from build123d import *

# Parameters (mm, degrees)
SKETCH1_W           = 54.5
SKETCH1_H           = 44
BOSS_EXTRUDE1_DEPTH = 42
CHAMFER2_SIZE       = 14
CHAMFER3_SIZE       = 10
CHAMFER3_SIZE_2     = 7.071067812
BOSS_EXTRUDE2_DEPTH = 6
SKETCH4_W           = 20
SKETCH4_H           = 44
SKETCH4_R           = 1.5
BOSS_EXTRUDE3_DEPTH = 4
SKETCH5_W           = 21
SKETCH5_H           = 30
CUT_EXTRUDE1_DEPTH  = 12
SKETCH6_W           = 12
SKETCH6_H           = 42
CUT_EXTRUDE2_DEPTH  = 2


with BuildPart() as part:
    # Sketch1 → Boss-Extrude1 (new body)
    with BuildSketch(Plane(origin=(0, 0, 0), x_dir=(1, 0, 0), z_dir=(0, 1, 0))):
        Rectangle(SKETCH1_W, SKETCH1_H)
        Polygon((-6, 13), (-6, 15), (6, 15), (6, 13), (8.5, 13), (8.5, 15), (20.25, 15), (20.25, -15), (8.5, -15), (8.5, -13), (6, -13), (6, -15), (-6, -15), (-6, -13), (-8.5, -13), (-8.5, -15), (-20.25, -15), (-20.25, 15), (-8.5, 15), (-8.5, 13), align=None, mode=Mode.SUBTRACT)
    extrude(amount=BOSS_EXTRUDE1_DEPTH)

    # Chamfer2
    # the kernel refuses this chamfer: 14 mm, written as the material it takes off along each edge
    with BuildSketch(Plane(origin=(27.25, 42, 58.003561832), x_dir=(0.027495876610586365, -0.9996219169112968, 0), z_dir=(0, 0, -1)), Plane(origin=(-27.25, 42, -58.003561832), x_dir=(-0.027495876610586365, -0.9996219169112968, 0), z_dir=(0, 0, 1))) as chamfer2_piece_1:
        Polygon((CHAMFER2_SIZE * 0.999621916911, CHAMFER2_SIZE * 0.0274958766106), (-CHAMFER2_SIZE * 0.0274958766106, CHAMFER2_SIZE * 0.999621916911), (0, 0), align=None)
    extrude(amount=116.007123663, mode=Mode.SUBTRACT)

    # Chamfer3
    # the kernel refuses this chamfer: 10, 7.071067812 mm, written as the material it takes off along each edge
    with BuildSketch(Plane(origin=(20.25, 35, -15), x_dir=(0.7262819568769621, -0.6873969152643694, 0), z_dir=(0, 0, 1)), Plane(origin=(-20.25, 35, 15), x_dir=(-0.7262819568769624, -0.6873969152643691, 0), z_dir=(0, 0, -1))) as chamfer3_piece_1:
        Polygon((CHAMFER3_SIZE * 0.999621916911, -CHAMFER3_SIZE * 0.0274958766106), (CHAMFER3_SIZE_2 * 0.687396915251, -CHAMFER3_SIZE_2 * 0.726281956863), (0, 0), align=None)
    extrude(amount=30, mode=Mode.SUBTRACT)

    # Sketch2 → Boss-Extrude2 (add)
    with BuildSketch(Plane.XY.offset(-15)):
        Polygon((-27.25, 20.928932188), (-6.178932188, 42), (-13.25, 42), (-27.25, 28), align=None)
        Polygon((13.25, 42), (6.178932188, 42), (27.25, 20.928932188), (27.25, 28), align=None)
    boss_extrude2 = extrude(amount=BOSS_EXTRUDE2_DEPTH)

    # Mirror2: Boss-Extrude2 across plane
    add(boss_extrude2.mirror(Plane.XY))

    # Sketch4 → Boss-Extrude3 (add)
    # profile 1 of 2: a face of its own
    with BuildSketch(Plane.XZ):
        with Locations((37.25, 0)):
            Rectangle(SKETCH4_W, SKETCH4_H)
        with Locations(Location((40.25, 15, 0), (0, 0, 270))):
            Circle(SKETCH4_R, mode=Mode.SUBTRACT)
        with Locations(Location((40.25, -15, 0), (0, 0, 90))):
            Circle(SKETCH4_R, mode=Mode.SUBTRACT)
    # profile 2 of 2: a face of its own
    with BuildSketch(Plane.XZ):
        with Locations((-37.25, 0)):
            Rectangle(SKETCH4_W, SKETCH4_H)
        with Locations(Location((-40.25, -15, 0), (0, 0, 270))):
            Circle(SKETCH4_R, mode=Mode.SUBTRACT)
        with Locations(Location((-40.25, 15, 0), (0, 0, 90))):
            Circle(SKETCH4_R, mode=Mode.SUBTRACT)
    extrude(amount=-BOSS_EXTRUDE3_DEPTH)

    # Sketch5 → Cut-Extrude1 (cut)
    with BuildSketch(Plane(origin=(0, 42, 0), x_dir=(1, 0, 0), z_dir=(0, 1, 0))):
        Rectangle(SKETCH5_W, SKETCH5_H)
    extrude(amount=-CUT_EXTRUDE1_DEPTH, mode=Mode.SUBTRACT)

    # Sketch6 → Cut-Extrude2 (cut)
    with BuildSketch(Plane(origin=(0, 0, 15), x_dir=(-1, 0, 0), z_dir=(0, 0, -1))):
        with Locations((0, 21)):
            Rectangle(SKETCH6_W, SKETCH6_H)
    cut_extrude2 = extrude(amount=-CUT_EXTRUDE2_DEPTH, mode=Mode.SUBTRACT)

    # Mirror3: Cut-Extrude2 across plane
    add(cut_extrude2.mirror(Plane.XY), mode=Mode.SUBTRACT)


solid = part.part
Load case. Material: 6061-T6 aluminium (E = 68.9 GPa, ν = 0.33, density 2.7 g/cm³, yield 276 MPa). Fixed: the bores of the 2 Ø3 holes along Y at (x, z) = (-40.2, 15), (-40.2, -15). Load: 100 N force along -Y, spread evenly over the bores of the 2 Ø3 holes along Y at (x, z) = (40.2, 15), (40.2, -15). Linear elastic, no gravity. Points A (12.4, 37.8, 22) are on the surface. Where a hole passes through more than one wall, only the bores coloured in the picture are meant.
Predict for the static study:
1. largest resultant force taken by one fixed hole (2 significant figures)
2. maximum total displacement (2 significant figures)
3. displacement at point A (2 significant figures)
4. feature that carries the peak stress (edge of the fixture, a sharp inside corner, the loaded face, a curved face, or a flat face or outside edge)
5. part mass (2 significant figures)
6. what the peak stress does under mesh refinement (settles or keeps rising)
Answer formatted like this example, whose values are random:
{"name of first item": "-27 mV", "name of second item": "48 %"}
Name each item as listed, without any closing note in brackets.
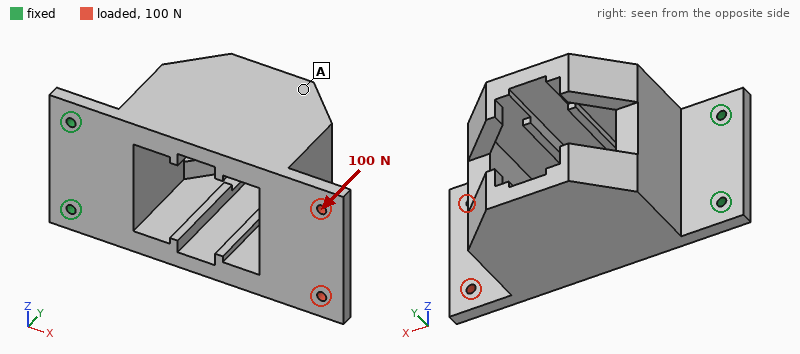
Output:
{"largest resultant force taken by one fixed hole": "65 N", "maximum total displacement": "0.63 mm", "displacement at point A": "0.44 mm", "feature that carries the peak stress": "edge of the fixture", "part mass": "130 g", "what the peak stress does under mesh refinement": "keeps rising"}
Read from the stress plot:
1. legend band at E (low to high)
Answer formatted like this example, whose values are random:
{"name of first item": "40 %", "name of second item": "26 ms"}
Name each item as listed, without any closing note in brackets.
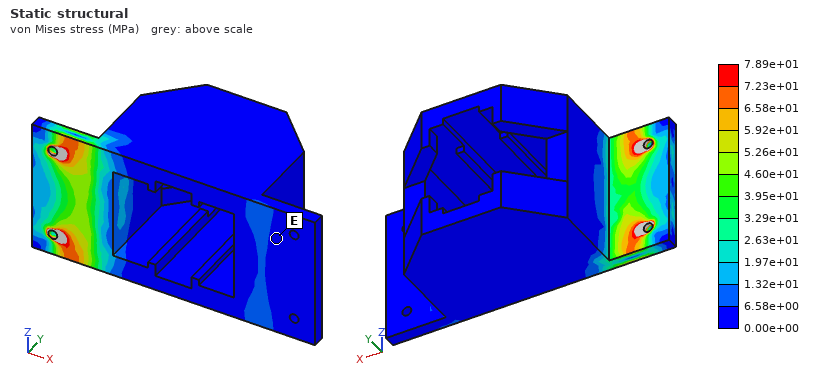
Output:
{"legend band at E": "0.00e+00 to 6.58e+00 MPa"}
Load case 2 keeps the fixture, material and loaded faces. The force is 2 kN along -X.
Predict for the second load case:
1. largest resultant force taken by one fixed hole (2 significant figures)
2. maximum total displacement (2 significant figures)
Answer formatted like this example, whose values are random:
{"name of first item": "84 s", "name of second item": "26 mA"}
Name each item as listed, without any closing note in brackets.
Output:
{"largest resultant force taken by one fixed hole": "1.0 kN", "maximum total displacement": "67 µm"}
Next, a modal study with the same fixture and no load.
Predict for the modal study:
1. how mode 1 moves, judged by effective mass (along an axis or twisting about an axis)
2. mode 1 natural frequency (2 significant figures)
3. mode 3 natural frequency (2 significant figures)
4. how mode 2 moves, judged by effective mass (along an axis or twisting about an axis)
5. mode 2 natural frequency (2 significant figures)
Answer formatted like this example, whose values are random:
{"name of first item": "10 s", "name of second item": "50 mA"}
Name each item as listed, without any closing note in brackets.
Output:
{"how mode 1 moves, judged by effective mass": "along Y", "mode 1 natural frequency": "310 Hz", "mode 3 natural frequency": "1700 Hz", "how mode 2 moves, judged by effective mass": "along Z", "mode 2 natural frequency": "1400 Hz"}
